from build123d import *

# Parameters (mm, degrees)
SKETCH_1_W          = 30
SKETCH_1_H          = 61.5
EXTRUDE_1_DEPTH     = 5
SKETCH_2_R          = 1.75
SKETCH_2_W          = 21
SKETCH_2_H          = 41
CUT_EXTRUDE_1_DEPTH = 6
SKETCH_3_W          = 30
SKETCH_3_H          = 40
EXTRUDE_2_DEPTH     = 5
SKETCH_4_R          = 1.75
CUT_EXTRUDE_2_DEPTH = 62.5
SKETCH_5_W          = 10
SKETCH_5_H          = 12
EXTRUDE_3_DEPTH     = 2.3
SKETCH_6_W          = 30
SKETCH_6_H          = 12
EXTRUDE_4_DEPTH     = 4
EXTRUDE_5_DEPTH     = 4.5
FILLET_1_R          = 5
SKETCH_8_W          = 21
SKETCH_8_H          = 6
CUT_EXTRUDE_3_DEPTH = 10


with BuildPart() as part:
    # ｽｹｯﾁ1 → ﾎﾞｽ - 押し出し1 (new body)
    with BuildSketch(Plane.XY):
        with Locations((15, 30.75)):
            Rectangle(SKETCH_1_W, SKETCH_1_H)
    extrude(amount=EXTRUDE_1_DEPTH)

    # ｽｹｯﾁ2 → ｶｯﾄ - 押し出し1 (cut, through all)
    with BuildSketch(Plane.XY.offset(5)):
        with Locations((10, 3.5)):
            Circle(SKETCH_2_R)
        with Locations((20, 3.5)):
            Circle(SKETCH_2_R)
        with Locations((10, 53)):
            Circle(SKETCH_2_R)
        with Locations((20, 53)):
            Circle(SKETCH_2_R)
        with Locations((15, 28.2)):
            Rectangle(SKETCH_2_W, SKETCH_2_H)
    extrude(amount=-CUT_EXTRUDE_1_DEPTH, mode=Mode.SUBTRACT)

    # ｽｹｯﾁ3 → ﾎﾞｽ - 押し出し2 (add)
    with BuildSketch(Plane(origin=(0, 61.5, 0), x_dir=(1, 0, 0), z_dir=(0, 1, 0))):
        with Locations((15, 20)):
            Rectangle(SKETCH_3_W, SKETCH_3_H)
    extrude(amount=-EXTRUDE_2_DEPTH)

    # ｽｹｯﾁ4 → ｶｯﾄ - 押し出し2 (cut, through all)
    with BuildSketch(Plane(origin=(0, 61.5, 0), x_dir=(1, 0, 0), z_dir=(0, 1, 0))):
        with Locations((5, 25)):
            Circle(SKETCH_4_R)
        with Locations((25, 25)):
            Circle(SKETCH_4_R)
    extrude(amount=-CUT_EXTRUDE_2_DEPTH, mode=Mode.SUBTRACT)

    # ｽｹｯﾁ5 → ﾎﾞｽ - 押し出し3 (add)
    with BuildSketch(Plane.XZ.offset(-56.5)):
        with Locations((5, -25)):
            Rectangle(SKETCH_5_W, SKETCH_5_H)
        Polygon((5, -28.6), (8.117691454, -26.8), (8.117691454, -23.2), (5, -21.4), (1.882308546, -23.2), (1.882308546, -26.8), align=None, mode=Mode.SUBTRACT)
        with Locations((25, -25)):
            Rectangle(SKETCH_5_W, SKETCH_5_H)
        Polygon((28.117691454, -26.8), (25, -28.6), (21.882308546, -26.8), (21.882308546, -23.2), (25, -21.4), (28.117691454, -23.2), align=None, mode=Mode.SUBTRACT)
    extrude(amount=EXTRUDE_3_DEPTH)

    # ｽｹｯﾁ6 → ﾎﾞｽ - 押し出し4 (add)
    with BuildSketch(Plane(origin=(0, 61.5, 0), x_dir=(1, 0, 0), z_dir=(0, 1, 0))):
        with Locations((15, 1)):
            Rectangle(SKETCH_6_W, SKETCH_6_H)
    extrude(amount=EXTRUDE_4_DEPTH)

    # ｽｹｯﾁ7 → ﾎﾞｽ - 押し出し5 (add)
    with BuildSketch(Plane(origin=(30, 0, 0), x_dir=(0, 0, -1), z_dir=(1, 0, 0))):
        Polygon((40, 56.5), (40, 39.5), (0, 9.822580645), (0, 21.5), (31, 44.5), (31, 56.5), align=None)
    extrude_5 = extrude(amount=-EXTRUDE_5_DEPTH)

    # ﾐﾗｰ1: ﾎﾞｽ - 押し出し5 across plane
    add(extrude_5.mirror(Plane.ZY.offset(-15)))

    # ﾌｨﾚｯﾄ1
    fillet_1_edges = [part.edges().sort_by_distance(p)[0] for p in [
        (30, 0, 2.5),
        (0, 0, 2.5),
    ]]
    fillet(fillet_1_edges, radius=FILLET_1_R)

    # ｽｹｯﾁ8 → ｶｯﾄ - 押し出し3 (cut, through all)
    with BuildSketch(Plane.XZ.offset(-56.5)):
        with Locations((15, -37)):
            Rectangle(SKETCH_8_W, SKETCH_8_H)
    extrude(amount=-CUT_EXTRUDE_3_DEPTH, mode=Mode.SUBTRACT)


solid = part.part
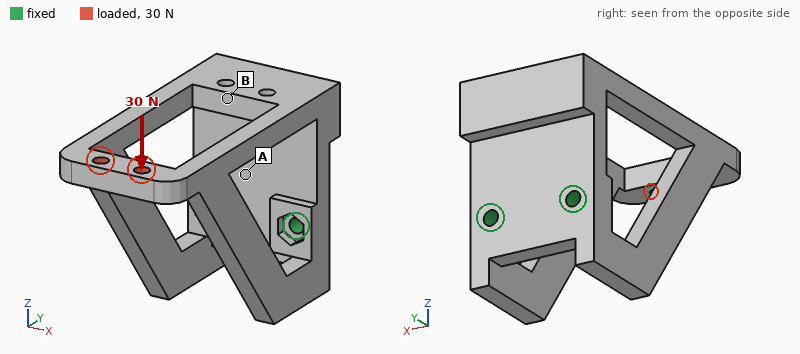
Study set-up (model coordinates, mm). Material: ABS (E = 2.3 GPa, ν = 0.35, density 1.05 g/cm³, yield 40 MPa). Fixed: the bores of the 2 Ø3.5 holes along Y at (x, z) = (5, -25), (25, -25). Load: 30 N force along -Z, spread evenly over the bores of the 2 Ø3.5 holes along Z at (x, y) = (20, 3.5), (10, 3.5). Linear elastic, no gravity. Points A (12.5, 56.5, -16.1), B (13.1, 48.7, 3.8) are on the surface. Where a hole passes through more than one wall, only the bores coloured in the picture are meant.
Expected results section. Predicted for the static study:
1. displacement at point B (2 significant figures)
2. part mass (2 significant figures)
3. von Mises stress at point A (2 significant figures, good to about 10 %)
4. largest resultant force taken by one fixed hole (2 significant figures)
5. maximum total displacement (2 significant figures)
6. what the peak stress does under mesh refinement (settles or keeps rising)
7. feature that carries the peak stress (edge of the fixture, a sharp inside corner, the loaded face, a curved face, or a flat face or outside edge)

0.33 mm
18 g
3.3 MPa
15 N
0.80 mm
keeps rising
edge of the fixture
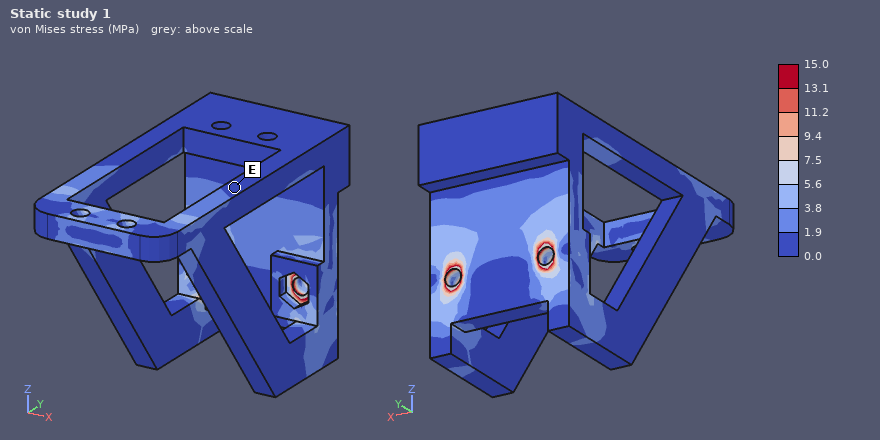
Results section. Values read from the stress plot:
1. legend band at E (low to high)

0.0 to 1.9 MPa
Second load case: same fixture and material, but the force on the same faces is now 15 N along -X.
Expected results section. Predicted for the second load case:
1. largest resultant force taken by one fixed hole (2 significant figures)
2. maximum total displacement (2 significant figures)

39 N
0.84 mm
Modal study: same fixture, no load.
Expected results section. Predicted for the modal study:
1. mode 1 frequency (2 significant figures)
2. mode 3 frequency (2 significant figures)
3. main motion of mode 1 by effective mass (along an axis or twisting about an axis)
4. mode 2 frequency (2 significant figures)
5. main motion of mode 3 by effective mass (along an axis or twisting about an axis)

410 Hz
1100 Hz
along X
500 Hz
twisting about Y
